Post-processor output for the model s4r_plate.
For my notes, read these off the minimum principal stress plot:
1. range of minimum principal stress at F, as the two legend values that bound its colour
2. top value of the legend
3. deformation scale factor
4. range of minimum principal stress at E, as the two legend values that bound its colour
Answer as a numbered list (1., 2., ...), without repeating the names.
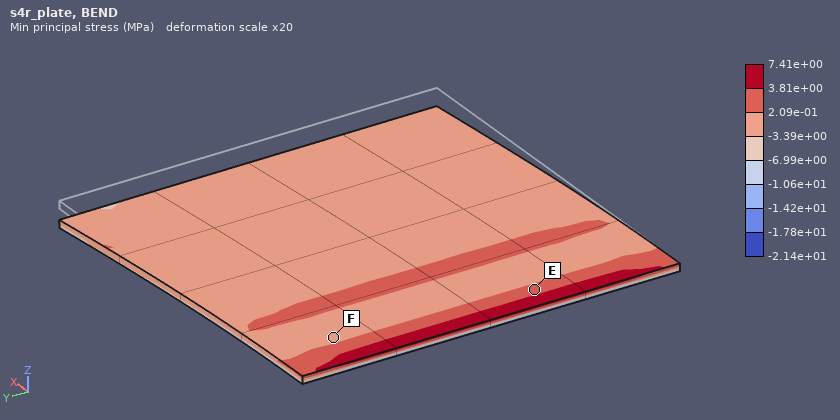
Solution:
1. -3.39e+00 to 2.09e-01 MPa
2. 7.41e+00 MPa
3. 20
4. 2.09e-01 to 3.81e+00 MPa
